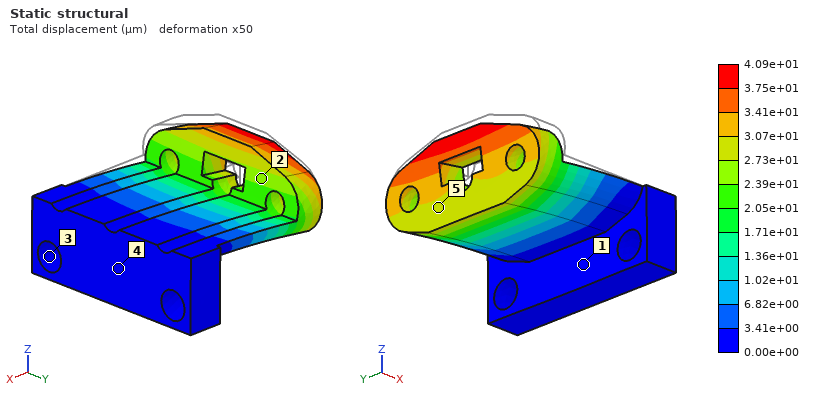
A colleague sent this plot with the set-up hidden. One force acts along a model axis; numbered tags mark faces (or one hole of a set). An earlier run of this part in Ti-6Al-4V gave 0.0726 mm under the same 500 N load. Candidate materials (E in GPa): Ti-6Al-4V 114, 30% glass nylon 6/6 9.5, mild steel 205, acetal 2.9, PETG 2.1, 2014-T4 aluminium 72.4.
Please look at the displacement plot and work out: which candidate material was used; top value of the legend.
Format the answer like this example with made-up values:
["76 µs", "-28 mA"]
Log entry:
["mild steel", "4.09e+01 µm"]
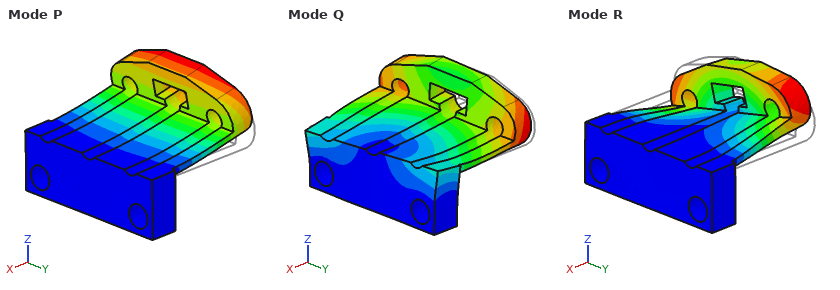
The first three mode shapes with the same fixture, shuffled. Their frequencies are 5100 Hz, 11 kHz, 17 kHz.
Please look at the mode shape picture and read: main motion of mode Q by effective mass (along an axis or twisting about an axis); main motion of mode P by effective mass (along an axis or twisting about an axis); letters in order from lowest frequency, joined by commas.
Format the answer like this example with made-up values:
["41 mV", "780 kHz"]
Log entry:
["along Y", "along Z", "P, R, Q"]
